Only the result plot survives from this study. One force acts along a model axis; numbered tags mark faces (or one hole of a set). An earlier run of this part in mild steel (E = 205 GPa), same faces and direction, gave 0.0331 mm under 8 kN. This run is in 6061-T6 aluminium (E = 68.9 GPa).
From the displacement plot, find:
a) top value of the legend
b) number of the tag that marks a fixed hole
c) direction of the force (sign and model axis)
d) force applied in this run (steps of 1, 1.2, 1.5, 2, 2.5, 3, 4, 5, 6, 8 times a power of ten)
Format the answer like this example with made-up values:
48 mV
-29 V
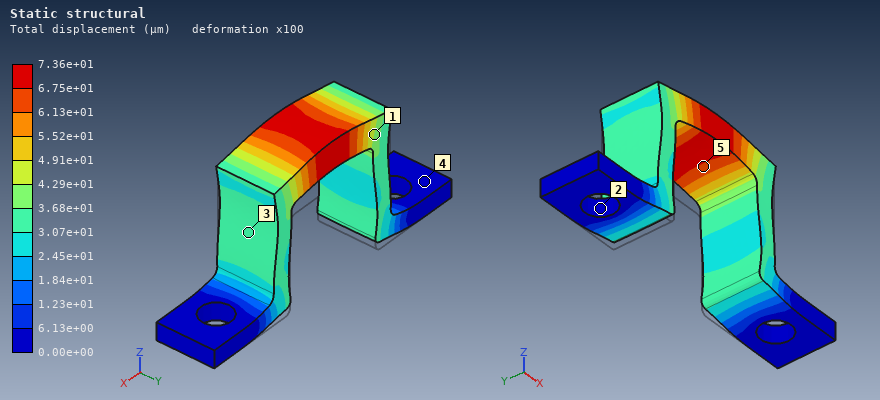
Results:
7.36e+01 µm
2
+Z
6 kN
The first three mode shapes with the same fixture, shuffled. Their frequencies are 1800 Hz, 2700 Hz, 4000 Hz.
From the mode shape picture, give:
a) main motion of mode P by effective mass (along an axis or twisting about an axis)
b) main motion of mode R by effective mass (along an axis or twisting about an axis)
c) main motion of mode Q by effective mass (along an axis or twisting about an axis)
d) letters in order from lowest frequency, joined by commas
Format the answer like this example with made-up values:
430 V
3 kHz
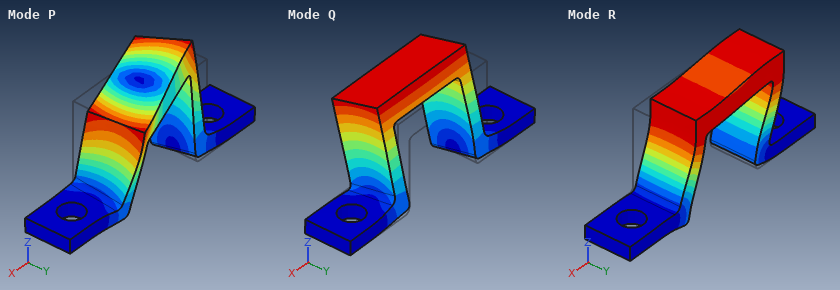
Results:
twisting about Z
along X
along Y
Q, R, P
